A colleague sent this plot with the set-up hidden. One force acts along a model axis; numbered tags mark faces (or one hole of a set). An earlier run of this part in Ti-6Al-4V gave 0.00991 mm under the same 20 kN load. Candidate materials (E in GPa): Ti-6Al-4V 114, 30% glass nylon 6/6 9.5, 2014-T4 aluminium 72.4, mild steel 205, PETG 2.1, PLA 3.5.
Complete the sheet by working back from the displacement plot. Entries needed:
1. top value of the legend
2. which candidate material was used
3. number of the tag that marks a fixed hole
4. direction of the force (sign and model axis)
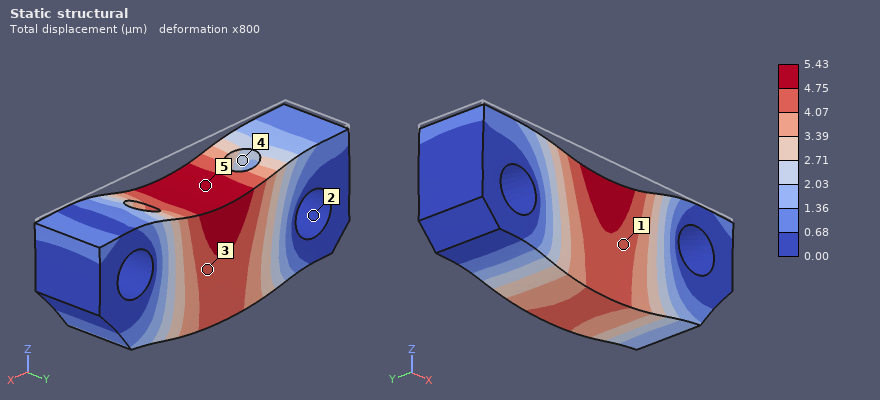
5.43 µm
mild steel
2
-Z
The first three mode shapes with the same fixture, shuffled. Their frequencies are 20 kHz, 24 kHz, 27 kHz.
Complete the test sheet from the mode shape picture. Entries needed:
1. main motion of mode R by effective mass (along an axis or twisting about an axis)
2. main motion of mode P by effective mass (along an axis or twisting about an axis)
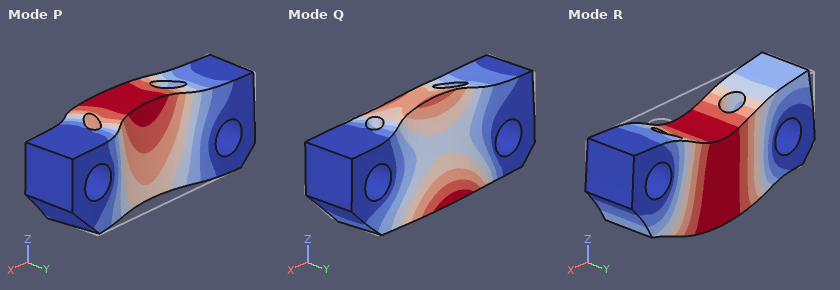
along Z
along Y
